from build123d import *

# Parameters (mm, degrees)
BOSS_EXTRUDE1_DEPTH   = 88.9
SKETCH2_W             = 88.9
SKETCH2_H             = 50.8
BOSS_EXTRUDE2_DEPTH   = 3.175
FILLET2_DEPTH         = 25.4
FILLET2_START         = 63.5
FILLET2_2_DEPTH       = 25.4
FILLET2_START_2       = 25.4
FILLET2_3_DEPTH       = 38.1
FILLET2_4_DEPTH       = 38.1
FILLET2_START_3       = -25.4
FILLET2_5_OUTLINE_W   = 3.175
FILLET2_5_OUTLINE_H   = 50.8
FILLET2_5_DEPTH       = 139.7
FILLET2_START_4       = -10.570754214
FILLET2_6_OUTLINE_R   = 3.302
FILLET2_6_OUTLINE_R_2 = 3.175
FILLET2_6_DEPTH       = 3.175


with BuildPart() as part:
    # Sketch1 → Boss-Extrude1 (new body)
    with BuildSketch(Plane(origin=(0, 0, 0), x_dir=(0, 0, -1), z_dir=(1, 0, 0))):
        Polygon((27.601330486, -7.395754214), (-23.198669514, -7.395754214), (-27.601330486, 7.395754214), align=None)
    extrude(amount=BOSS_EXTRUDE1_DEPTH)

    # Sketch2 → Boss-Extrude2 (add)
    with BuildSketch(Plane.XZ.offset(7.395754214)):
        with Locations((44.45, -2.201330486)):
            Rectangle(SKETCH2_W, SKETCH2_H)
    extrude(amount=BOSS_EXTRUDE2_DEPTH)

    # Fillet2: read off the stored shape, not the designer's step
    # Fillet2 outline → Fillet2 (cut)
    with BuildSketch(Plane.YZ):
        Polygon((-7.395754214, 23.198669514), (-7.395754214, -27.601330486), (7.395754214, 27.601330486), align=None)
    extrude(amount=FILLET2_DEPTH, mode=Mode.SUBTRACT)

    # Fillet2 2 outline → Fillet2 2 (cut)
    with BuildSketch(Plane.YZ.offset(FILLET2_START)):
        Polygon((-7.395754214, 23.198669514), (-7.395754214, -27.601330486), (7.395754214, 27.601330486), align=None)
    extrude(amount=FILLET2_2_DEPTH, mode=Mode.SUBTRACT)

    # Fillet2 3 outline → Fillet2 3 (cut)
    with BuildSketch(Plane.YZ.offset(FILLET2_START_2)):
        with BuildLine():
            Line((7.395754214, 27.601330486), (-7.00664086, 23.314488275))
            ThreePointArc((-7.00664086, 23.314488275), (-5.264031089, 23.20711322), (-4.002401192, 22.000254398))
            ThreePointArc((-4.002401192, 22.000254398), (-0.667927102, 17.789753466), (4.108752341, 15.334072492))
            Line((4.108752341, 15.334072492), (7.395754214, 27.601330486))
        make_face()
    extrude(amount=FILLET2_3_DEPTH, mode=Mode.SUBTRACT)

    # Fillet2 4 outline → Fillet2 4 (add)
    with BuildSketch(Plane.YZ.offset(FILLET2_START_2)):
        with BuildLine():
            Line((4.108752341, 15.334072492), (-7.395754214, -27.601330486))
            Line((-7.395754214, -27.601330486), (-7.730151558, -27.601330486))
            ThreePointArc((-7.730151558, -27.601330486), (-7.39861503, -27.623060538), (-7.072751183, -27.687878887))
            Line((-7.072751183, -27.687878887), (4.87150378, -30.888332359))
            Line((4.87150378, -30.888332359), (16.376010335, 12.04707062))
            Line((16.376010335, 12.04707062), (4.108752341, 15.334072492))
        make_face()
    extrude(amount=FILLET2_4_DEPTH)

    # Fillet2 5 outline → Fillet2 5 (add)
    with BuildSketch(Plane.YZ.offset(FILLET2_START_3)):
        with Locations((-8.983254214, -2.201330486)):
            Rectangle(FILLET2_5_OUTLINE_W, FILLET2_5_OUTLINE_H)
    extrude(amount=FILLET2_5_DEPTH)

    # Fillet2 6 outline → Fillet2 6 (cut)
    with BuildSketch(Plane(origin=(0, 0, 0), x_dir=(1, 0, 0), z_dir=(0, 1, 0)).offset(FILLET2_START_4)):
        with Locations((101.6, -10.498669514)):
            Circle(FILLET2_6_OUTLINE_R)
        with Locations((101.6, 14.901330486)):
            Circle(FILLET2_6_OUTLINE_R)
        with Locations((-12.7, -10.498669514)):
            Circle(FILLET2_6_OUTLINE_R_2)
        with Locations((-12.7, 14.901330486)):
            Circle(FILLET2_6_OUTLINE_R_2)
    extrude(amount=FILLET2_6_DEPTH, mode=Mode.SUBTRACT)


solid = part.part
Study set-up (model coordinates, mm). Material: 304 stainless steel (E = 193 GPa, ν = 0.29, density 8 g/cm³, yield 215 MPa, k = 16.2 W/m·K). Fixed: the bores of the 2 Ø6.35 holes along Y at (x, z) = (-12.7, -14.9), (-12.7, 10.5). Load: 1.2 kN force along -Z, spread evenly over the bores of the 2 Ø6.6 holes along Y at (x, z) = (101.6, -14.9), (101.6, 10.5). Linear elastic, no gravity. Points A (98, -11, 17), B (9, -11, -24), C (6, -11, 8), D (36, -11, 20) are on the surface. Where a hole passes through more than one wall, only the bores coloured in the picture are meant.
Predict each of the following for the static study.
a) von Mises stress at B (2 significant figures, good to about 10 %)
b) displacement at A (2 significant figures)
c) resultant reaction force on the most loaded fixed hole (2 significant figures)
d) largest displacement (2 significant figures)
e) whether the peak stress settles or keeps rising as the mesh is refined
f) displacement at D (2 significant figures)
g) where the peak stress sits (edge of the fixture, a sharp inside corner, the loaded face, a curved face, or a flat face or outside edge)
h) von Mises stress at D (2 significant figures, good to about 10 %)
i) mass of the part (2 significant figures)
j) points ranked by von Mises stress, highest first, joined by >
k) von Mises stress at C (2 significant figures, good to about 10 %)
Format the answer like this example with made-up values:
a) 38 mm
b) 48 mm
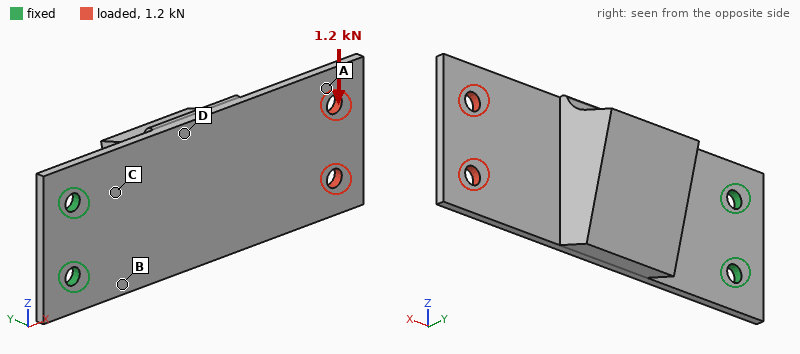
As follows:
a) 64 MPa
b) 0.11 mm
c) 4.7 kN
d) 0.13 mm
e) keeps rising
f) 0.040 mm
g) edge of the fixture
h) 29 MPa
i) 440 g
j) B > C > D > A
k) 48 MPa
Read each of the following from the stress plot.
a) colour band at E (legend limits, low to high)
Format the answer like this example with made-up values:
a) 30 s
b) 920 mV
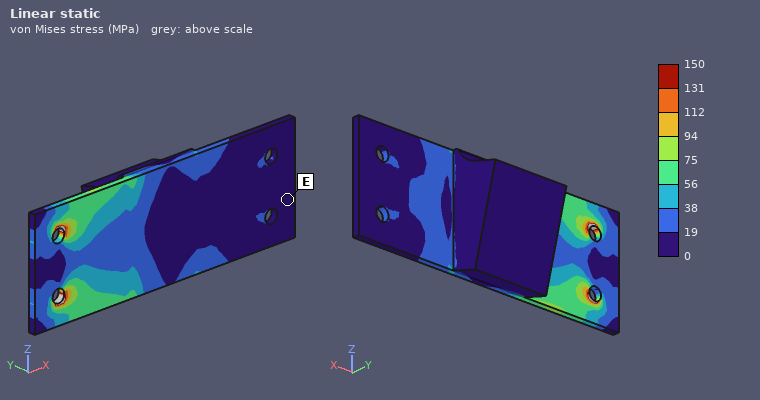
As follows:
a) 0 to 19 MPa
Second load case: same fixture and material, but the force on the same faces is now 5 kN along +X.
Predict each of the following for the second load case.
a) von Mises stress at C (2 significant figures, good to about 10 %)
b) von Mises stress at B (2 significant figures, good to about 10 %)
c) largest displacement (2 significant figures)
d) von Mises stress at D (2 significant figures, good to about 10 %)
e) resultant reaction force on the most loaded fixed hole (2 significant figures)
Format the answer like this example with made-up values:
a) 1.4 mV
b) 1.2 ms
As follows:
a) 34 MPa
b) 28 MPa
c) 44 µm
d) 21 MPa
e) 2.5 kN
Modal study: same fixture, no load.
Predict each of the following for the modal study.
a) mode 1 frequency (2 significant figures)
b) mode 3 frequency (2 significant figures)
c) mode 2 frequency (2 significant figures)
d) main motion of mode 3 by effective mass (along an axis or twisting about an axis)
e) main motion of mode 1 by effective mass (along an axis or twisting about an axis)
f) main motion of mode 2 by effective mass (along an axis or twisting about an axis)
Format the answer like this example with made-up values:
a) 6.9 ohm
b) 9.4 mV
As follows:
a) 140 Hz
b) 990 Hz
c) 690 Hz
d) along Y
e) along Y
f) along Z
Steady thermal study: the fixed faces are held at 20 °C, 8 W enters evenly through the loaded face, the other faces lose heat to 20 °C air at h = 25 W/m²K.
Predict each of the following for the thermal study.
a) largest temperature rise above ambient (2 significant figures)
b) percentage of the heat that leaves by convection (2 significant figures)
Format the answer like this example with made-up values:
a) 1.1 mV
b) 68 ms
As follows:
a) 74 K
b) 96 %
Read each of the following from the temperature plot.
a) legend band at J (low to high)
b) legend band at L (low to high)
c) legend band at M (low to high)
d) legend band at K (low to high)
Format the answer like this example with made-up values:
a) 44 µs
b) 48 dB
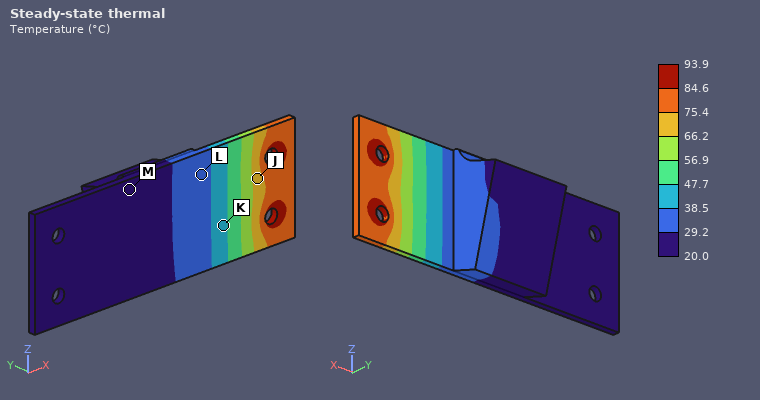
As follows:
a) 66.2 to 75.4 °C
b) 29.2 to 38.5 °C
c) 20.0 to 29.2 °C
d) 38.5 to 47.7 °C
